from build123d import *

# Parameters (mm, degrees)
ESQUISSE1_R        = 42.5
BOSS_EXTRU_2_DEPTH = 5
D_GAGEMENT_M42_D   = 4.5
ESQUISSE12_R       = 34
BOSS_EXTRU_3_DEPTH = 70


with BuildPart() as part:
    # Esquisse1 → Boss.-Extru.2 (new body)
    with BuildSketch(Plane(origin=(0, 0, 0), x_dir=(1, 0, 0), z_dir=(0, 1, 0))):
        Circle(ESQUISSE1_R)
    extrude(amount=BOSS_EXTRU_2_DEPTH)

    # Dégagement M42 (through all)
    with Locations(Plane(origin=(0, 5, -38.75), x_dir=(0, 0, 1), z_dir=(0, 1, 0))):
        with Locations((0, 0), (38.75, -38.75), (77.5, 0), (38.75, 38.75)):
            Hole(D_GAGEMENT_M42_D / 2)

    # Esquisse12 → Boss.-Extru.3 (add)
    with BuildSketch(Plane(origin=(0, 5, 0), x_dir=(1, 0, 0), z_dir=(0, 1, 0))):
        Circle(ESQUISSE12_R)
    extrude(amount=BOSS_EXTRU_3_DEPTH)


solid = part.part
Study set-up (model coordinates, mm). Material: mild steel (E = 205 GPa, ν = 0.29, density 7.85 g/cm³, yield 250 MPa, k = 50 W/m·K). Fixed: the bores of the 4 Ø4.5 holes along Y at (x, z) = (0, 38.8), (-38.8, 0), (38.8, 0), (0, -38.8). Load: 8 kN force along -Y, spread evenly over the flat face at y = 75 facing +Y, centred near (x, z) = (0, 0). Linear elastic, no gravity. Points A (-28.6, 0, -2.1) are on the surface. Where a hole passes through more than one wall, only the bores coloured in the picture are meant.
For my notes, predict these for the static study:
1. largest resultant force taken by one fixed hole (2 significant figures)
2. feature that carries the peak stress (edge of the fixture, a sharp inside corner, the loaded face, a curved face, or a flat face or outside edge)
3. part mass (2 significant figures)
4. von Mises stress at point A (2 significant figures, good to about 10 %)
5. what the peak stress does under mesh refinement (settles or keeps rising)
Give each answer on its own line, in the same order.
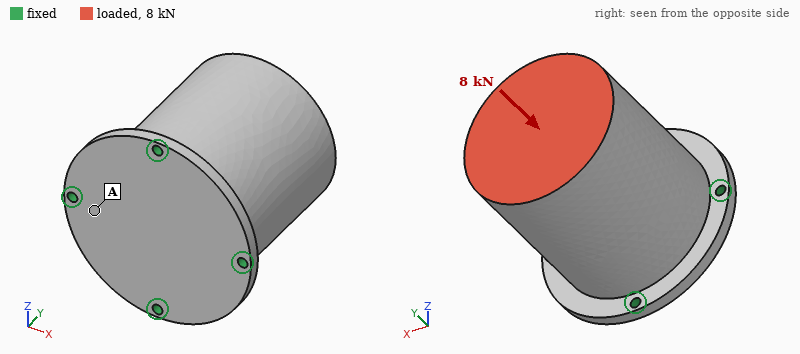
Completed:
2.2 kN
edge of the fixture
2.2 kg
18 MPa
keeps rising
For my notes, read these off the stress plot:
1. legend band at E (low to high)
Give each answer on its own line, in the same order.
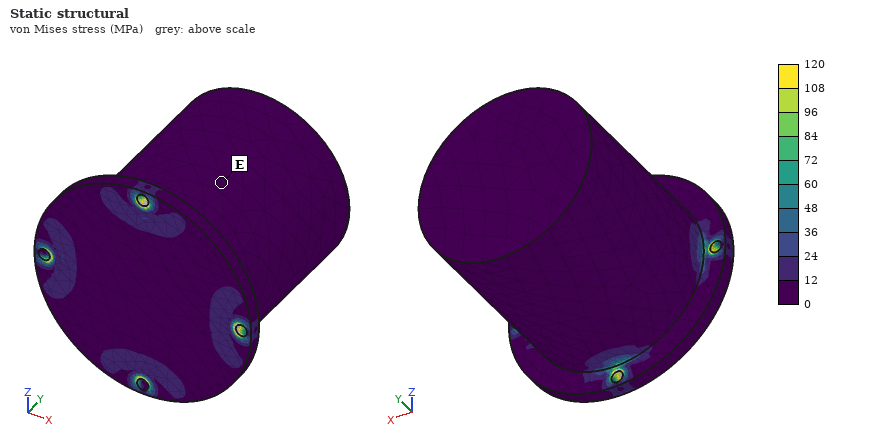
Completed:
0 to 12 MPa
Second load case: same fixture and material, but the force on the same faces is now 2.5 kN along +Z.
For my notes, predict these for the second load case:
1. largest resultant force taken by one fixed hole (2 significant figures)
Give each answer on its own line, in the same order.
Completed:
2.7 kN
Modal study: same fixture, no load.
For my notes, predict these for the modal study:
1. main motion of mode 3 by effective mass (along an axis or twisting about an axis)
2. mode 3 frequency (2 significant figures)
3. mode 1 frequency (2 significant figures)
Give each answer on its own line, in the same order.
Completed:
along Y
4400 Hz
2500 Hz
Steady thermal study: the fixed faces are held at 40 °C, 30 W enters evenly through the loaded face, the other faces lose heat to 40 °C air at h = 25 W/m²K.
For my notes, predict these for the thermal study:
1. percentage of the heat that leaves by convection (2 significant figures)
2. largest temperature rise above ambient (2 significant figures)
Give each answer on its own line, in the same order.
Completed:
25 %
21 K
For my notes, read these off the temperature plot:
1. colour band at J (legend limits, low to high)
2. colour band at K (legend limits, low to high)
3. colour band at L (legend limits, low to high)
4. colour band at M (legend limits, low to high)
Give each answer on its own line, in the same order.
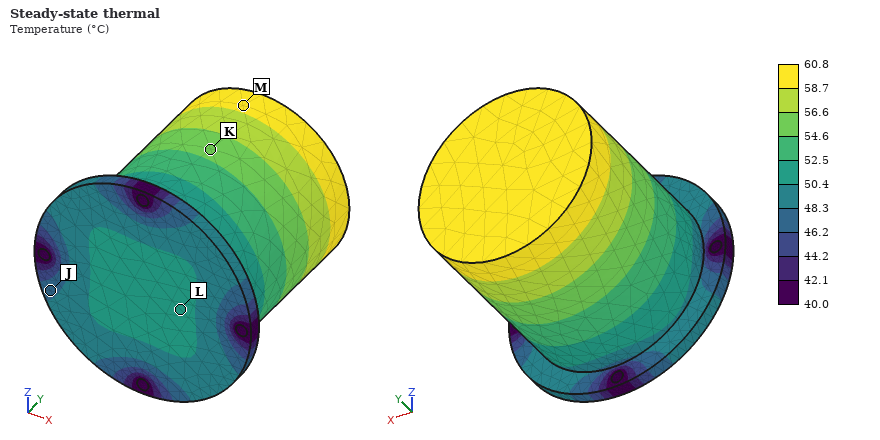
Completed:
46.2 to 48.3 °C
54.6 to 56.6 °C
50.4 to 52.5 °C
58.7 to 60.8 °C
